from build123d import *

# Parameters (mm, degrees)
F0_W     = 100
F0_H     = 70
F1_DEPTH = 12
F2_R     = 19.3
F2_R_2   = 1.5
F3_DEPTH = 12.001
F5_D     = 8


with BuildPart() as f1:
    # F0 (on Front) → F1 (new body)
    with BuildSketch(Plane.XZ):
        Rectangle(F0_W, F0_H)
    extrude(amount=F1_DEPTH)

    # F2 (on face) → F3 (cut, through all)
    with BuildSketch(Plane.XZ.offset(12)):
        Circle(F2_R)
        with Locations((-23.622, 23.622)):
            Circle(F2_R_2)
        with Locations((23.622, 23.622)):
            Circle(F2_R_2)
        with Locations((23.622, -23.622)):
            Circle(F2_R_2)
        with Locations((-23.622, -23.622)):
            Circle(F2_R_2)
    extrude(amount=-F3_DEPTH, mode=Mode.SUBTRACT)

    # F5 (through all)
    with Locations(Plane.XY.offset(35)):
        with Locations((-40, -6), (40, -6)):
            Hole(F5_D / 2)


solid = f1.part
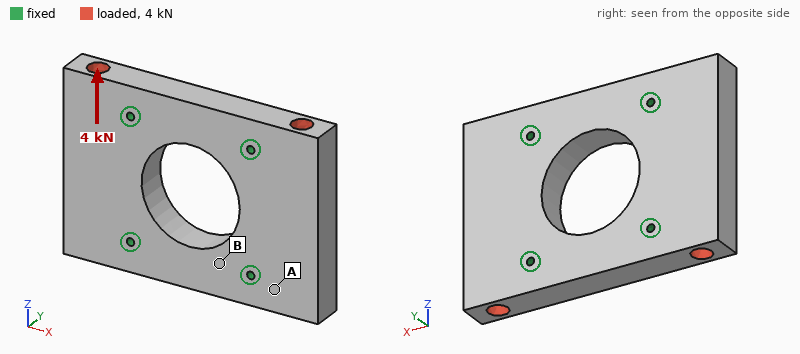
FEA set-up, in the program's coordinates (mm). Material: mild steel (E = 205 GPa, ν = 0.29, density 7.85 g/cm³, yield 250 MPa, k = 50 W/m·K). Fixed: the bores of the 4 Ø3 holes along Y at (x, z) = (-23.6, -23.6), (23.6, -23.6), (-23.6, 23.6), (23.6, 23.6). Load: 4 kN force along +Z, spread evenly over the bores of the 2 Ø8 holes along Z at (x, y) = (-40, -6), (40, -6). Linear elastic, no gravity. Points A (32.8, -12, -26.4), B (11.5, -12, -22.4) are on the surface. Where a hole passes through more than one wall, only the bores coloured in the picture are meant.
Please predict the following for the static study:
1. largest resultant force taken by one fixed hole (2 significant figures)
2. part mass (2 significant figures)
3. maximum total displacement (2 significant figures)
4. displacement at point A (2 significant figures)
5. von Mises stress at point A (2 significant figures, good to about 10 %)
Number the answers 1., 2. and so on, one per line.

1. 1.1 kN
2. 490 g
3. 1.3 µm
4. 0.56 µm
5. 3.8 MPa
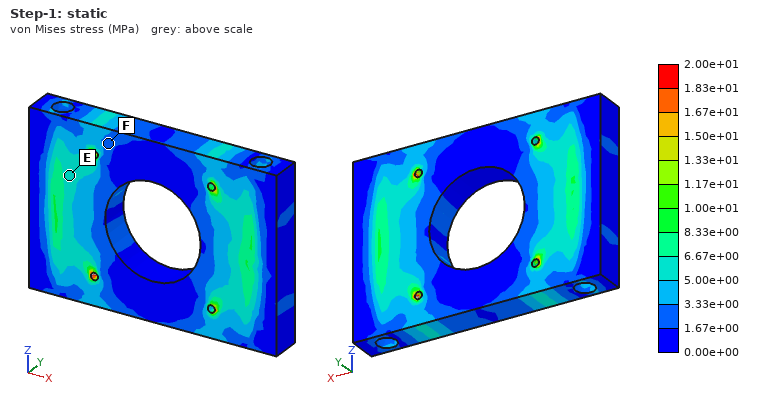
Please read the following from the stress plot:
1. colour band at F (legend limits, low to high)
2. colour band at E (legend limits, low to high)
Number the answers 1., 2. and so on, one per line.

1. 1.67e+00 to 3.33e+00 MPa
2. 5.00e+00 to 6.67e+00 MPa
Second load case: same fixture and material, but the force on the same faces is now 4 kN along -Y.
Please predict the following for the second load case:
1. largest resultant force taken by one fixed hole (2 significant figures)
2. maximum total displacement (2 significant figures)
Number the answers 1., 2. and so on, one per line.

1. 1.0 kN
2. 9.5 µm
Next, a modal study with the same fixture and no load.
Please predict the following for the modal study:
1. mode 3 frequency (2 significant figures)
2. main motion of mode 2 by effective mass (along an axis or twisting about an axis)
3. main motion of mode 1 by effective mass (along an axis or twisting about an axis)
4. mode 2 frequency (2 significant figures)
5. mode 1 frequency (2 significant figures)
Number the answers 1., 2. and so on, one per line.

1. 13 kHz
2. twisting about Z
3. along Y
4. 8700 Hz
5. 8300 Hz
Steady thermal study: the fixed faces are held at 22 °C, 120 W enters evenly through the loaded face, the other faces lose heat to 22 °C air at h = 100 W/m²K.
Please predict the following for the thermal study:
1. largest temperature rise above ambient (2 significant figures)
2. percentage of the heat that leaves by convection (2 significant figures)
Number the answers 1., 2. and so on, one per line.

1. 37 K
2. 26 %
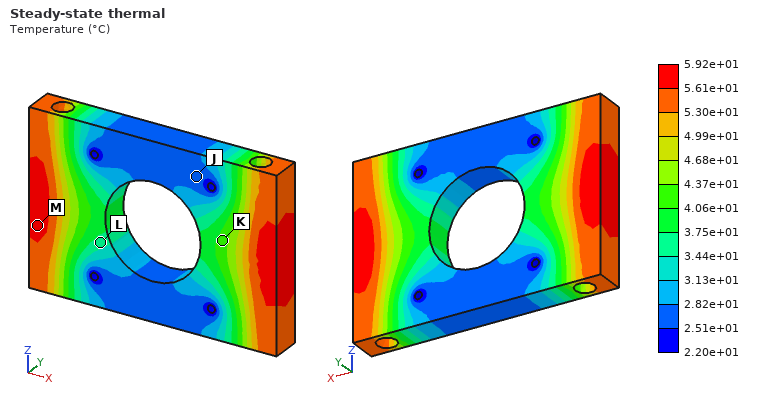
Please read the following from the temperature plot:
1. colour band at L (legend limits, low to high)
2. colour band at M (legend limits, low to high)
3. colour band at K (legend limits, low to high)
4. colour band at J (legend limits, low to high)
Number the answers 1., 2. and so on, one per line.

1. 3.44e+01 to 3.75e+01 °C
2. 5.61e+01 to 5.92e+01 °C
3. 4.06e+01 to 4.37e+01 °C
4. 2.51e+01 to 2.82e+01 °C
